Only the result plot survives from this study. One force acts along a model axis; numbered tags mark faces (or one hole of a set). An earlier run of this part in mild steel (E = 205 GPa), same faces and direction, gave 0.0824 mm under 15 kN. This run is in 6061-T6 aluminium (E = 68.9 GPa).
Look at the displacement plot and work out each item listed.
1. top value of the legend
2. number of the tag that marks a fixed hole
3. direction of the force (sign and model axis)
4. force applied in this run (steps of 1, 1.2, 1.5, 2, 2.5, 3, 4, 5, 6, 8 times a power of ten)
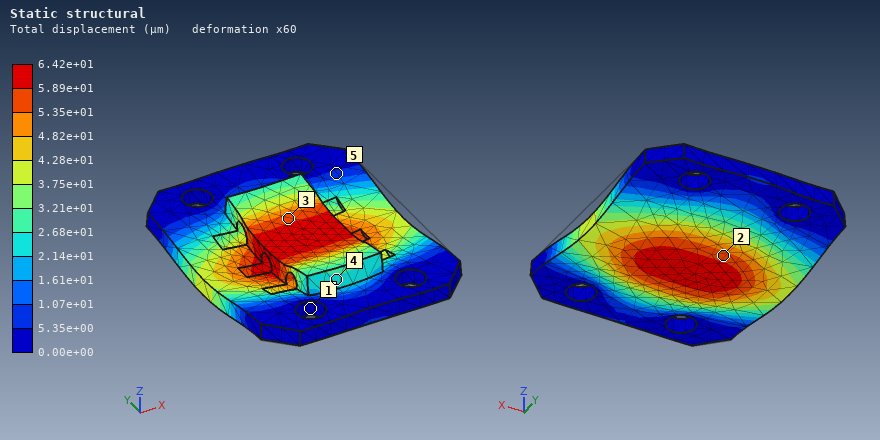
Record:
6.42e+01 µm
1
-Z
4 kN
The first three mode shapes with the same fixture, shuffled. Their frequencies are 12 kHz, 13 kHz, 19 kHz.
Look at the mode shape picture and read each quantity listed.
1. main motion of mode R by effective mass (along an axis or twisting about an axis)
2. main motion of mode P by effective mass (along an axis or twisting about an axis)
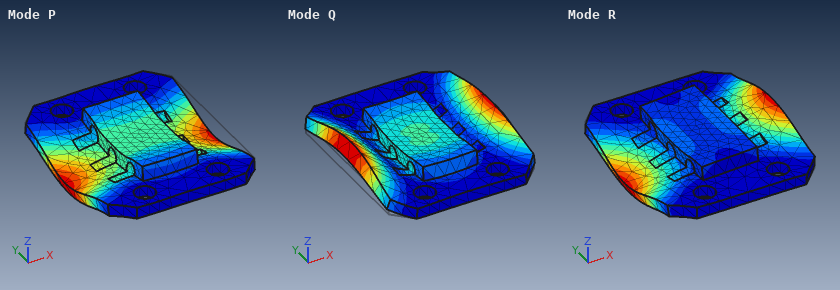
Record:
twisting about Y
along Z
